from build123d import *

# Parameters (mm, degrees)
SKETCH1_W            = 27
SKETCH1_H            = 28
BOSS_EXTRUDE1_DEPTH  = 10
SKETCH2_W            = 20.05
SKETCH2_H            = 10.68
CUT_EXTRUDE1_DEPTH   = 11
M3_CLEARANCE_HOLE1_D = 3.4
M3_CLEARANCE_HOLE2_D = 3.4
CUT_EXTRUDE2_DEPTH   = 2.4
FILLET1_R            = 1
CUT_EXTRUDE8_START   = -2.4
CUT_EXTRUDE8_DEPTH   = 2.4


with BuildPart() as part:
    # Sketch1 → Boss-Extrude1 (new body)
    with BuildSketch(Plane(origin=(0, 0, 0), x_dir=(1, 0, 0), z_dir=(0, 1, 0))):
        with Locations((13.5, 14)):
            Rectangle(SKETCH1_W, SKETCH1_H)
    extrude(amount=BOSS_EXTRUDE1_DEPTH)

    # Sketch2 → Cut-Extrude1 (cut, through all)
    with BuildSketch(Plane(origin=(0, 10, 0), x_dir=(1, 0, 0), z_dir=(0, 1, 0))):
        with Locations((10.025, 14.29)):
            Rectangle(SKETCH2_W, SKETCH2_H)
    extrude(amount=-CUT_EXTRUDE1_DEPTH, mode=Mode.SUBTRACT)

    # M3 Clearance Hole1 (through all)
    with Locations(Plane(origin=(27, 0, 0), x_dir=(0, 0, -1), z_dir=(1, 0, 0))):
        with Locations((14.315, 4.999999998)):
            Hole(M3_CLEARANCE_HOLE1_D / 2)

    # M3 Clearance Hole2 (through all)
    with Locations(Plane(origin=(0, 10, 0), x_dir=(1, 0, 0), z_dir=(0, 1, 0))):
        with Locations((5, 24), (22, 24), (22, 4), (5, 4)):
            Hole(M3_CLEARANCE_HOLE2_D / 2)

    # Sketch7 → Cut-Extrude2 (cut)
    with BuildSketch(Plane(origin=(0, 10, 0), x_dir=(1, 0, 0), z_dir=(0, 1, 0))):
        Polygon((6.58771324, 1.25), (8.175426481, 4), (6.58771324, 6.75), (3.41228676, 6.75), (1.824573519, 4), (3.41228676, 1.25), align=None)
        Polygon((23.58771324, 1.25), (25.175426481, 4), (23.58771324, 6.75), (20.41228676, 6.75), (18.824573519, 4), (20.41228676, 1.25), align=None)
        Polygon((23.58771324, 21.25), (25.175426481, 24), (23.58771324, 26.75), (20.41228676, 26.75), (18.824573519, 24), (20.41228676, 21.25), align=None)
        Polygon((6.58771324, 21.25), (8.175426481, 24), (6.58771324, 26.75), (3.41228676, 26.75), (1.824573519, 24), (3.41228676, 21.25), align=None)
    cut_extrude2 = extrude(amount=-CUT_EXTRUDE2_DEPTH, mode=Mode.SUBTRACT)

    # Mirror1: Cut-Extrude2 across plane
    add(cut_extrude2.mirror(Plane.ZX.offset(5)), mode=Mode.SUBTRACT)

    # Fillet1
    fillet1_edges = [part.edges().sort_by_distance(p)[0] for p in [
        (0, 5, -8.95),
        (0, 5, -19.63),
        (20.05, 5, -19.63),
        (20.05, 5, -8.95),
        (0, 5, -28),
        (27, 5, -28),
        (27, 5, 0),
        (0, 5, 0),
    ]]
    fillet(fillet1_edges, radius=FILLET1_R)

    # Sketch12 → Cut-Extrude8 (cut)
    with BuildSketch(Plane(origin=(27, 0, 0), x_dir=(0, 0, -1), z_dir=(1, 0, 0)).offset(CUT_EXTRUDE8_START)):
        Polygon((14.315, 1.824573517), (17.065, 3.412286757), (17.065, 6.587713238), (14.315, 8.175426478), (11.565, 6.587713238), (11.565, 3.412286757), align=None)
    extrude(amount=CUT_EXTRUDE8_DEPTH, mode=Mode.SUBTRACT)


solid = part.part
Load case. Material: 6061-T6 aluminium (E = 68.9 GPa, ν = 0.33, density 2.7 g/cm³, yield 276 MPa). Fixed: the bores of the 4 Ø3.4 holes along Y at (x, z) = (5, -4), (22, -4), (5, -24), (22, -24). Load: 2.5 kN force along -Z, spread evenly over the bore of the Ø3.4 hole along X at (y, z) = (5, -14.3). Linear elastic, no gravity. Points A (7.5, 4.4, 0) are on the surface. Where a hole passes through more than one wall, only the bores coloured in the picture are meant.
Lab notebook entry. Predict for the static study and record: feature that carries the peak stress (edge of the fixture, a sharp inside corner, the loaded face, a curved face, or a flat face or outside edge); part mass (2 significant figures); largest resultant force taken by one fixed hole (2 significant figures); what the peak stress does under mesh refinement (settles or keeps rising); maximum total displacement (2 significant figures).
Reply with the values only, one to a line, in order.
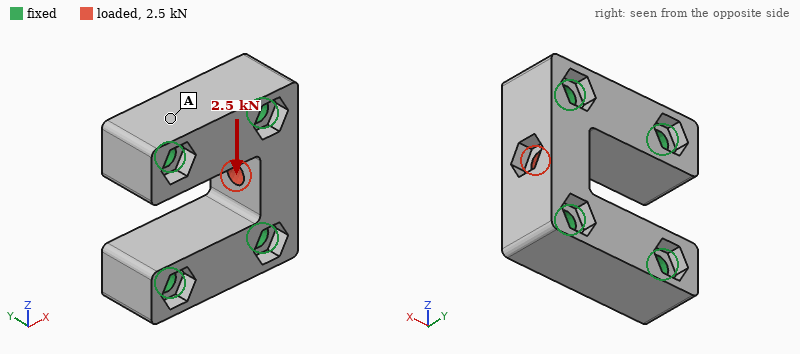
a sharp inside corner
12 g
1.3 kN
keeps rising
4.8 µm
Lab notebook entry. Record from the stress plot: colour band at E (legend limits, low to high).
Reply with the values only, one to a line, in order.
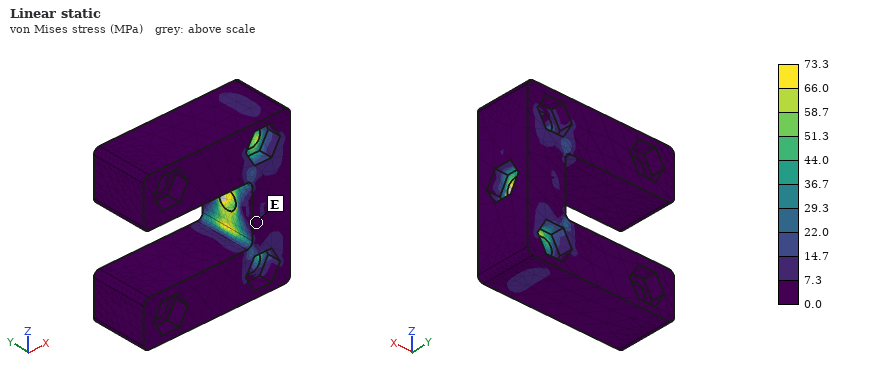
0.0 to 7.3 MPa
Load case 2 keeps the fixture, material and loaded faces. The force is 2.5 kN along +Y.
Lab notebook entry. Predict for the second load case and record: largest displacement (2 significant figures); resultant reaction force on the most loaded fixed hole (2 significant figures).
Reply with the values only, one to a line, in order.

14 µm
1.3 kN
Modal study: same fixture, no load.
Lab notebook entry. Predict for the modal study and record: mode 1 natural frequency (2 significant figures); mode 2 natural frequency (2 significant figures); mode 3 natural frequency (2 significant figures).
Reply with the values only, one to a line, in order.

54 kHz
56 kHz
61 kHz
